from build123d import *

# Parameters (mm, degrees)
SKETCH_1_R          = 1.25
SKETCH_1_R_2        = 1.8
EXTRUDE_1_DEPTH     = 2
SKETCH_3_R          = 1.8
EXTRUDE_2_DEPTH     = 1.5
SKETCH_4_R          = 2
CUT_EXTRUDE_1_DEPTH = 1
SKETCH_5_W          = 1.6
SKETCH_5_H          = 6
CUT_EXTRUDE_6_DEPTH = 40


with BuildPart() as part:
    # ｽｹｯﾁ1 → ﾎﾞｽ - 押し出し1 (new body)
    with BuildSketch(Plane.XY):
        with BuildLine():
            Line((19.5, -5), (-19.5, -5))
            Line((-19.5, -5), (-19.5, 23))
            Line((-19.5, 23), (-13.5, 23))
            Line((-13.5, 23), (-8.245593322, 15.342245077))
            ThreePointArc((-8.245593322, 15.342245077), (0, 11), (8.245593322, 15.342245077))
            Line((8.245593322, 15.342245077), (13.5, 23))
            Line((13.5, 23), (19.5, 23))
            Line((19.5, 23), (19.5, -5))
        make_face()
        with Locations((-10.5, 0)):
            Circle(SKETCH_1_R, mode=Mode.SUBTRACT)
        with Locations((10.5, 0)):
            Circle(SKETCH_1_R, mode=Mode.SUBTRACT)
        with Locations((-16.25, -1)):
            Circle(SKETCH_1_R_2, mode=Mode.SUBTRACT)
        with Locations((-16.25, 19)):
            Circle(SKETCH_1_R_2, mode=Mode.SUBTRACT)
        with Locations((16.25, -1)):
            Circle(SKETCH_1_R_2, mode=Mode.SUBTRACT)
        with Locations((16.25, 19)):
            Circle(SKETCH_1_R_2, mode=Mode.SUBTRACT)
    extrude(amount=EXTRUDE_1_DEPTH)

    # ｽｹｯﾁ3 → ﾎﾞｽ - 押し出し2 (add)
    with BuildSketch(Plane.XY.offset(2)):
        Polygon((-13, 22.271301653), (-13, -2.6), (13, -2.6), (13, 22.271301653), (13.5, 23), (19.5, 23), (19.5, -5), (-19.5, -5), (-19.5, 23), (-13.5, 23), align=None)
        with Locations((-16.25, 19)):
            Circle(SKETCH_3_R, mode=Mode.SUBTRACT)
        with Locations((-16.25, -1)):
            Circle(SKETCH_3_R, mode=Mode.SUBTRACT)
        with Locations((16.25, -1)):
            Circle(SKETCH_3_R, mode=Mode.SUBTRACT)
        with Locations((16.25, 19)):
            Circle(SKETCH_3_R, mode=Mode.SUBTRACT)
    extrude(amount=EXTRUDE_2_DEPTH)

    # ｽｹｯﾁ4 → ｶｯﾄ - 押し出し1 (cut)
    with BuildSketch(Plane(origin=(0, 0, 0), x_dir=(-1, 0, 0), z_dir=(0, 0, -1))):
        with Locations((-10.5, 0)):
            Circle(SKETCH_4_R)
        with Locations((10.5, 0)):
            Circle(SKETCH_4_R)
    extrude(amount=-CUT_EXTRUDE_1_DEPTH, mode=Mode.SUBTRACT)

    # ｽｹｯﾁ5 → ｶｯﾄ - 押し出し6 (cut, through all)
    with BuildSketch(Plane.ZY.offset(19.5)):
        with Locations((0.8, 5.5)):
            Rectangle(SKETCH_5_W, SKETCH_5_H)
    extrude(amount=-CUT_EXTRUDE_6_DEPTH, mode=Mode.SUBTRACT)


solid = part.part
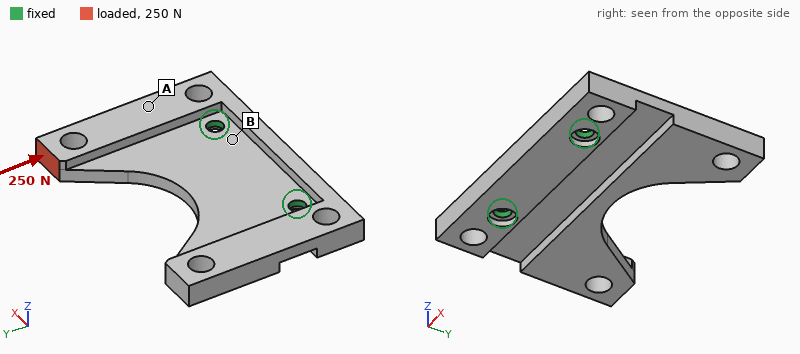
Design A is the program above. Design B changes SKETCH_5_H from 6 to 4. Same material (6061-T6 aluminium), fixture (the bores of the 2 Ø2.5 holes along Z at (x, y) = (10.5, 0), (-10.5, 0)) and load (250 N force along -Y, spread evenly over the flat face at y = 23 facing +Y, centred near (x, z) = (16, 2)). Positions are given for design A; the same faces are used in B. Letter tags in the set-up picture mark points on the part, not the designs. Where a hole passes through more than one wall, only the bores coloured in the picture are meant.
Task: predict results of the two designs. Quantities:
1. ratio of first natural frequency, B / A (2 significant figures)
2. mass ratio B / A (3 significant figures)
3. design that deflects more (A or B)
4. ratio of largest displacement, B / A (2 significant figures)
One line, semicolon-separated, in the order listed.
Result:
1.1; 1.07; A; 0.74
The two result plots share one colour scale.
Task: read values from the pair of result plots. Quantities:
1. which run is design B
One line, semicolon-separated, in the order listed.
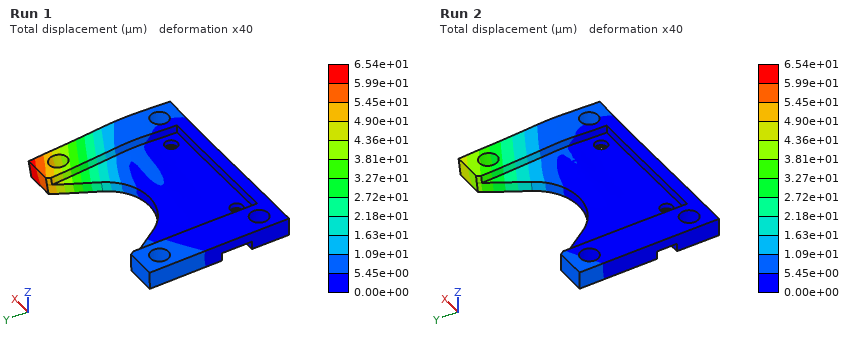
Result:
Run 2
